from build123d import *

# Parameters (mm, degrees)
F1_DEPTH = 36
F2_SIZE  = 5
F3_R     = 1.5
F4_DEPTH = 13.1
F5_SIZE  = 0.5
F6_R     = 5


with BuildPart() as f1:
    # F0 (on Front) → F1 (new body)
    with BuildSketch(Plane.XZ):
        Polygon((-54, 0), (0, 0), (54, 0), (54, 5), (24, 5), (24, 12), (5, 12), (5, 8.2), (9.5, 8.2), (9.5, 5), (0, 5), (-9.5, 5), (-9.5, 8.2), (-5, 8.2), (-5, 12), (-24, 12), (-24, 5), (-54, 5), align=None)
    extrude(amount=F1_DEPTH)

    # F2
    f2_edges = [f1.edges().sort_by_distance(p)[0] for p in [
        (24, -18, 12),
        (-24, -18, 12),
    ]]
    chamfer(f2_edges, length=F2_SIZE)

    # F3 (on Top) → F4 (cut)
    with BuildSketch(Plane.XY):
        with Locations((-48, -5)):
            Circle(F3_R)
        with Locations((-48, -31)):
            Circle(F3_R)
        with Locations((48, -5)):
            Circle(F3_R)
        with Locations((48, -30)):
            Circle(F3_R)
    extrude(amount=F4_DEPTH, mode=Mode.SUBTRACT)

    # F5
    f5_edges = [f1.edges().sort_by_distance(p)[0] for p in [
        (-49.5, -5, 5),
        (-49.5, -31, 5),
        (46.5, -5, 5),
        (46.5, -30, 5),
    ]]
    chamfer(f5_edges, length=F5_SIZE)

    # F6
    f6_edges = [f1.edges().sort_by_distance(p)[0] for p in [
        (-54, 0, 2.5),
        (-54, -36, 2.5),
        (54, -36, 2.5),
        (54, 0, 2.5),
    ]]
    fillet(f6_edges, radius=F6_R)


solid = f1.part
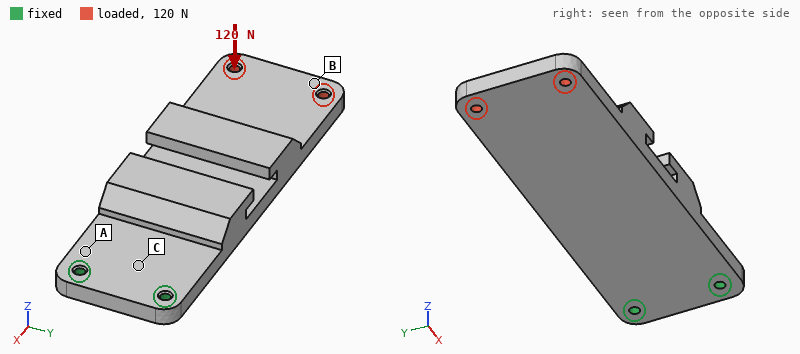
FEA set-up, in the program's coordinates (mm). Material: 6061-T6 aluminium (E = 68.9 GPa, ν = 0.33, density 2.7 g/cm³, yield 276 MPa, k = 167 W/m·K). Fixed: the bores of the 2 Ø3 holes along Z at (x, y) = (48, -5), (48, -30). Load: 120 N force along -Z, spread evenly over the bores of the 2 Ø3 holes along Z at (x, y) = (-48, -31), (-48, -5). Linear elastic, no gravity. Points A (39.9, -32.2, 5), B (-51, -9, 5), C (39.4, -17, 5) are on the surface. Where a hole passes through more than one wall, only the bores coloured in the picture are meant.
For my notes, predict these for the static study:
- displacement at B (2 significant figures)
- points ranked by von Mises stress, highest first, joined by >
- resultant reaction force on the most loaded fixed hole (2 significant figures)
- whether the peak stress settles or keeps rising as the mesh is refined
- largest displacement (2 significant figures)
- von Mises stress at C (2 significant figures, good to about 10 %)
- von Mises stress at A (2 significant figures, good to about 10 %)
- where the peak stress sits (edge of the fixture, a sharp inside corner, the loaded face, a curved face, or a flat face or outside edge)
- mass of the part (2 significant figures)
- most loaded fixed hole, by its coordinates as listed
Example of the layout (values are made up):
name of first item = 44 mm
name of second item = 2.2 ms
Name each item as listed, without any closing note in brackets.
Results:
displacement at B = 1.2 mm
points ranked by von Mises stress, highest first, joined by > = A > C > B
resultant reaction force on the most loaded fixed hole = 65 N
whether the peak stress settles or keeps rising as the mesh is refined = keeps rising
largest displacement = 1.3 mm
von Mises stress at C = 58 MPa
von Mises stress at A = 74 MPa
where the peak stress sits = edge of the fixture
mass of the part = 72 g
most loaded fixed hole, by its coordinates as listed = (48, -30)
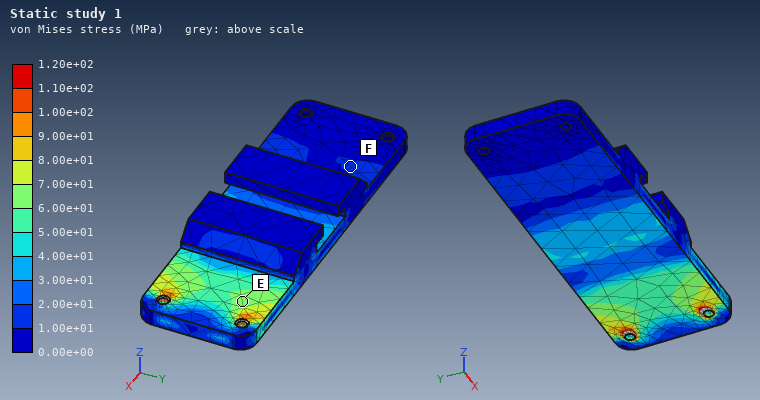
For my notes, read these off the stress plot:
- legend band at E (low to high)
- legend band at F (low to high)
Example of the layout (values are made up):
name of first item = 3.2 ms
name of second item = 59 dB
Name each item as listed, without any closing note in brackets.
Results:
legend band at E = 6.00e+01 to 7.00e+01 MPa
legend band at F = 1.00e+01 to 2.00e+01 MPa
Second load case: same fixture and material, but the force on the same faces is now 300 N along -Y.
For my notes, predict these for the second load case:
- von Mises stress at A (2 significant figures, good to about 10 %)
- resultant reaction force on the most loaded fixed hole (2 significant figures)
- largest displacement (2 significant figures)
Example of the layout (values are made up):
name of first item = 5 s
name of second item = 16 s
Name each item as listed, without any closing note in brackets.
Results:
von Mises stress at A = 21 MPa
resultant reaction force on the most loaded fixed hole = 1.1 kN
largest displacement = 83 µm
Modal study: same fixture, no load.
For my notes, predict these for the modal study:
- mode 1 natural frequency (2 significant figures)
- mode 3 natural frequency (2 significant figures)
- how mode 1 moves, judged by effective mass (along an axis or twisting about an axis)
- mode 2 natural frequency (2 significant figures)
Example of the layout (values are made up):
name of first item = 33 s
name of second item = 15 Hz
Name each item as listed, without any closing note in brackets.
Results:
mode 1 natural frequency = 370 Hz
mode 3 natural frequency = 2300 Hz
how mode 1 moves, judged by effective mass = along Z
mode 2 natural frequency = 2200 Hz
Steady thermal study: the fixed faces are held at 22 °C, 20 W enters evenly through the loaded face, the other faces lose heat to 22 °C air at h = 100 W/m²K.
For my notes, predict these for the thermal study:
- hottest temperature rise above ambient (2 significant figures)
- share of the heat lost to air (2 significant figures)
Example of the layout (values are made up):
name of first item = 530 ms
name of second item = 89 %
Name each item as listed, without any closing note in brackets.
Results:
hottest temperature rise above ambient = 34 K
share of the heat lost to air = 68 %
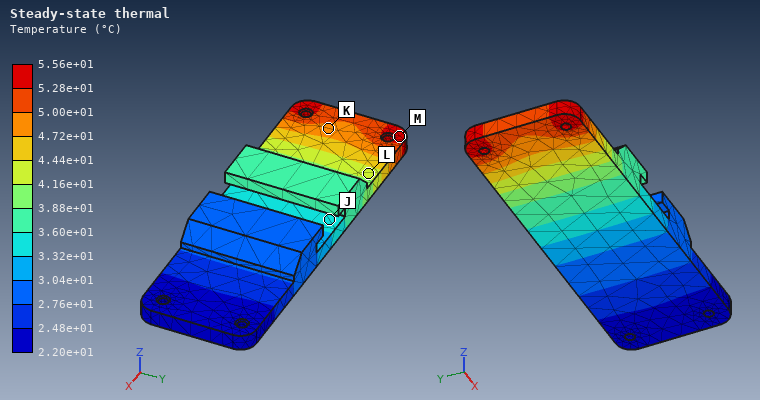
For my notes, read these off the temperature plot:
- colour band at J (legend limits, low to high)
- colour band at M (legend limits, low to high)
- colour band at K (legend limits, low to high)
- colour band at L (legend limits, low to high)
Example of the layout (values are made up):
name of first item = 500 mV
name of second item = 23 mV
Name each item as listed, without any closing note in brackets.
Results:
colour band at J = 3.32e+01 to 3.60e+01 °C
colour band at M = 5.28e+01 to 5.56e+01 °C
colour band at K = 4.72e+01 to 5.00e+01 °C
colour band at L = 4.16e+01 to 4.44e+01 °C
